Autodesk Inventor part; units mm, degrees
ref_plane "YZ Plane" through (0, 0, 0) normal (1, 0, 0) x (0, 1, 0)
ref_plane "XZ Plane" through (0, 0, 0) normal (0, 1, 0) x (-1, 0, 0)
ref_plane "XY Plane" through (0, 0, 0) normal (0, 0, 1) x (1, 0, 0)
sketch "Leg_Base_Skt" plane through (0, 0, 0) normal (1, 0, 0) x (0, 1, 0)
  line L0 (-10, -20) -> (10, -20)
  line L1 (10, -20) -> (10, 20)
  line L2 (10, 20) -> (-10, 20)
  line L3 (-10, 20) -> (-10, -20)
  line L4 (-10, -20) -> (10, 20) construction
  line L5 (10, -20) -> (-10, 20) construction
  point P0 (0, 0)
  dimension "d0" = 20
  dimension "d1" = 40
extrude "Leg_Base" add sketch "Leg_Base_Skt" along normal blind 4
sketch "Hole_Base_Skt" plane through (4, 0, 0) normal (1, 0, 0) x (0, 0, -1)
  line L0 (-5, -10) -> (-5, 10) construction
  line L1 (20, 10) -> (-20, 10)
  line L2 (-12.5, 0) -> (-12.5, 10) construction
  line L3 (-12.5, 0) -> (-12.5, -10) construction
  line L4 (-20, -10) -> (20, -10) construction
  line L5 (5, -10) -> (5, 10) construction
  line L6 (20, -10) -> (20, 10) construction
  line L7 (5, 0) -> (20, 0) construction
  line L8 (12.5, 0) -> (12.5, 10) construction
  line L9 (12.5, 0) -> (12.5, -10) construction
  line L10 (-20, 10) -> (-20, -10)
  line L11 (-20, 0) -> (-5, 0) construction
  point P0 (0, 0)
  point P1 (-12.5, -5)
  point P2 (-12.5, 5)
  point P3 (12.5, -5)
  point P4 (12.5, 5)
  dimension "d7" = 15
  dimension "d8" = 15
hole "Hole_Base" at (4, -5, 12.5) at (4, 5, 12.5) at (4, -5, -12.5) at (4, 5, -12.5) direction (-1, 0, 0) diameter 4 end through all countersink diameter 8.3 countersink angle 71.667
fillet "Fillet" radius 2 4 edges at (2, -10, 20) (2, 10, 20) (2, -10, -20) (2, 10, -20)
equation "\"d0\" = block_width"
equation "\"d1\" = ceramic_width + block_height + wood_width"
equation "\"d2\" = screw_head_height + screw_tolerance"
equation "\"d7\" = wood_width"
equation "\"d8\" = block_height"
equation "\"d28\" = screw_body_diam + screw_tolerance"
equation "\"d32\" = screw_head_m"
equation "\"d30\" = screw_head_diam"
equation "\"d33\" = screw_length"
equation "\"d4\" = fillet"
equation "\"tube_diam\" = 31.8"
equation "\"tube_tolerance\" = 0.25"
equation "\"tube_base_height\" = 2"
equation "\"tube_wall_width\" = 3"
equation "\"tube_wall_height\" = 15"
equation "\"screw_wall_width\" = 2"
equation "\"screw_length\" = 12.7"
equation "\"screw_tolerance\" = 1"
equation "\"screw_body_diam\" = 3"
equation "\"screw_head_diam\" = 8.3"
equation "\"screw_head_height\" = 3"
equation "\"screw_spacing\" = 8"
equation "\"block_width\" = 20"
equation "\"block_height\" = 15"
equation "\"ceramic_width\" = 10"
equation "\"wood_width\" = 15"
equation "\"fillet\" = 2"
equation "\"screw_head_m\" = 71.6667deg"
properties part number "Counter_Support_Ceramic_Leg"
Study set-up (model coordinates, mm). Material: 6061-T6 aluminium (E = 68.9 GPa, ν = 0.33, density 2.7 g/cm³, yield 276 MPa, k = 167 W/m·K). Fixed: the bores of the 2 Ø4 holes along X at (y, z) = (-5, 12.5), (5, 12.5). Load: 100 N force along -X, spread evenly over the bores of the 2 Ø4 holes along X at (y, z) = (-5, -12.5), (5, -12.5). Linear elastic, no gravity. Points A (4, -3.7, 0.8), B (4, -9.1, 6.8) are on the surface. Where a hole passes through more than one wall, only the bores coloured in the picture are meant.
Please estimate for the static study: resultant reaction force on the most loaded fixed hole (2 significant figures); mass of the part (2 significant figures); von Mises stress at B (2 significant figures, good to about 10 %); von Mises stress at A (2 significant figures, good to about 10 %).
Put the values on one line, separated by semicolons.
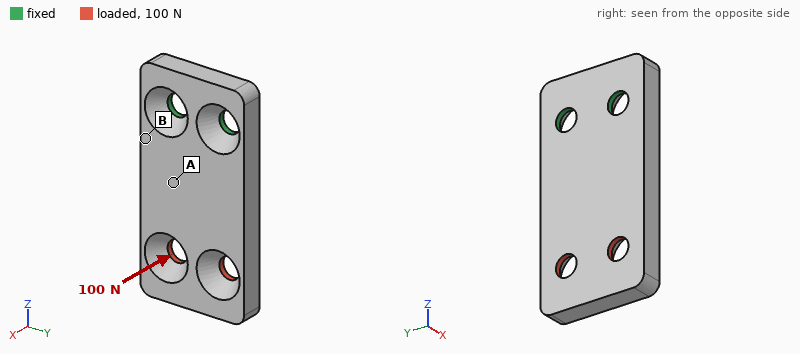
68 N; 7.5 g; 47 MPa; 23 MPa
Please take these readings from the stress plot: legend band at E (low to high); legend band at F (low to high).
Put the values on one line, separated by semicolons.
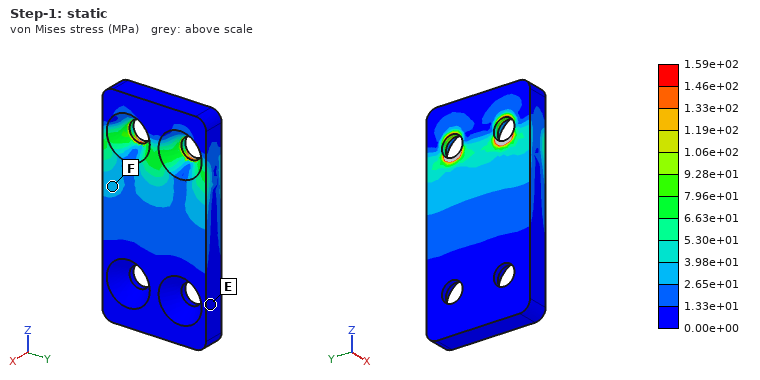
0.00e+00 to 1.33e+01 MPa; 2.65e+01 to 3.98e+01 MPa
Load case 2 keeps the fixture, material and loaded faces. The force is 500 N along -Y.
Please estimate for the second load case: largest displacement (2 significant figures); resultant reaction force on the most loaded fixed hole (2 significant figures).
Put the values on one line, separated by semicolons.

60 µm; 1.0 kN
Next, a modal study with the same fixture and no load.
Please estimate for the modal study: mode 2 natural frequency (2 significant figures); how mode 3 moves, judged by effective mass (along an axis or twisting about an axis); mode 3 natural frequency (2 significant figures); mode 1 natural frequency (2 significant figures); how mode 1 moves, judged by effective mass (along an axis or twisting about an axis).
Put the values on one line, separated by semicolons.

8900 Hz; along Y; 11 kHz; 2500 Hz; along X
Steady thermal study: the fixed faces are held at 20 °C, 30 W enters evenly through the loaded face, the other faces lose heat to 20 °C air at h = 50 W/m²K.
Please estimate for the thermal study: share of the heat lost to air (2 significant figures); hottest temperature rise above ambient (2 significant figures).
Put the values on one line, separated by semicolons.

11 %; 69 K
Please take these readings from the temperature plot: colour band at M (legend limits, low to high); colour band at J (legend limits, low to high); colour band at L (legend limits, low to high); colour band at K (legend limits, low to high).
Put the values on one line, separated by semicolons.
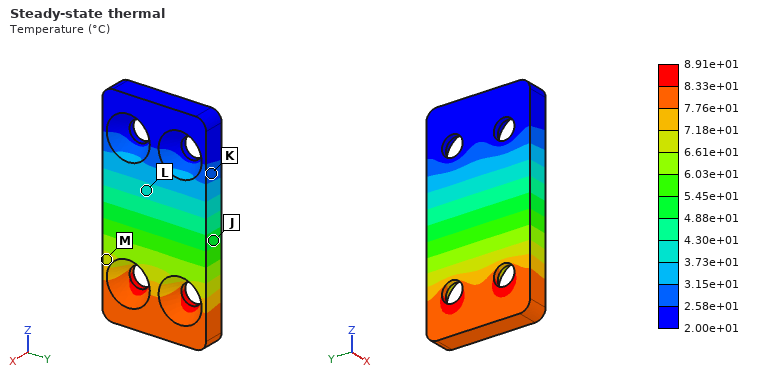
6.61e+01 to 7.18e+01 °C; 4.88e+01 to 5.45e+01 °C; 3.73e+01 to 4.30e+01 °C; 2.58e+01 to 3.15e+01 °C
